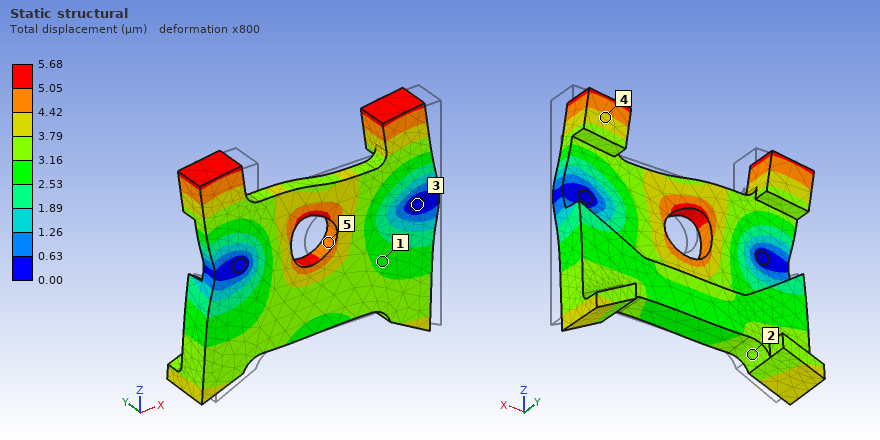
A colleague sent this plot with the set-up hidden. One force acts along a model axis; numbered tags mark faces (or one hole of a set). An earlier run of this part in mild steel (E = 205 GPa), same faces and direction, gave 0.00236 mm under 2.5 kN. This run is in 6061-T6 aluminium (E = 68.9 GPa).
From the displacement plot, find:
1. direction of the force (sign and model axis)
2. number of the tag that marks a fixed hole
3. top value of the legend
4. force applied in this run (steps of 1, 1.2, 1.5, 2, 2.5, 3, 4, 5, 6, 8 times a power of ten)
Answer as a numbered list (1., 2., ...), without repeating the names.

1. -X
2. 3
3. 5.68 µm
4. 2 kN
